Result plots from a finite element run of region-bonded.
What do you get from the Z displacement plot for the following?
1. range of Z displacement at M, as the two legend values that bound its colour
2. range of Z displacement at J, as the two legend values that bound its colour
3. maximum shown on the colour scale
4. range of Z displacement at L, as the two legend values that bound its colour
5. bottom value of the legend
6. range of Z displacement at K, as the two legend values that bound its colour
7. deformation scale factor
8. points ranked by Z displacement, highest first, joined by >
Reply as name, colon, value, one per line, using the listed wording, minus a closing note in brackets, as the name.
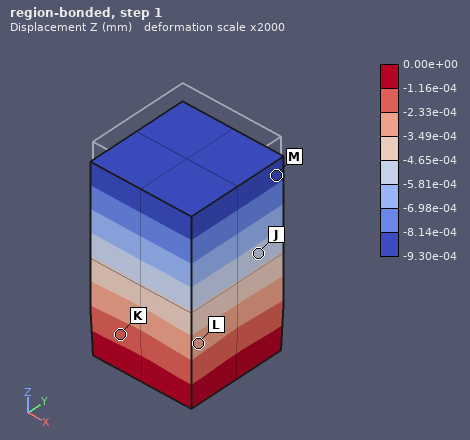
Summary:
range of Z displacement at M, as the two legend values that bound its colour: -9.30e-04 to -8.14e-04 mm
range of Z displacement at J, as the two legend values that bound its colour: -5.81e-04 to -4.65e-04 mm
maximum shown on the colour scale: 0.00e+00 mm
range of Z displacement at L, as the two legend values that bound its colour: -3.49e-04 to -2.33e-04 mm
bottom value of the legend: -9.30e-04 mm
range of Z displacement at K, as the two legend values that bound its colour: -2.33e-04 to -1.16e-04 mm
deformation scale factor: 2000
points ranked by Z displacement, highest first, joined by >: K > L > J > M
